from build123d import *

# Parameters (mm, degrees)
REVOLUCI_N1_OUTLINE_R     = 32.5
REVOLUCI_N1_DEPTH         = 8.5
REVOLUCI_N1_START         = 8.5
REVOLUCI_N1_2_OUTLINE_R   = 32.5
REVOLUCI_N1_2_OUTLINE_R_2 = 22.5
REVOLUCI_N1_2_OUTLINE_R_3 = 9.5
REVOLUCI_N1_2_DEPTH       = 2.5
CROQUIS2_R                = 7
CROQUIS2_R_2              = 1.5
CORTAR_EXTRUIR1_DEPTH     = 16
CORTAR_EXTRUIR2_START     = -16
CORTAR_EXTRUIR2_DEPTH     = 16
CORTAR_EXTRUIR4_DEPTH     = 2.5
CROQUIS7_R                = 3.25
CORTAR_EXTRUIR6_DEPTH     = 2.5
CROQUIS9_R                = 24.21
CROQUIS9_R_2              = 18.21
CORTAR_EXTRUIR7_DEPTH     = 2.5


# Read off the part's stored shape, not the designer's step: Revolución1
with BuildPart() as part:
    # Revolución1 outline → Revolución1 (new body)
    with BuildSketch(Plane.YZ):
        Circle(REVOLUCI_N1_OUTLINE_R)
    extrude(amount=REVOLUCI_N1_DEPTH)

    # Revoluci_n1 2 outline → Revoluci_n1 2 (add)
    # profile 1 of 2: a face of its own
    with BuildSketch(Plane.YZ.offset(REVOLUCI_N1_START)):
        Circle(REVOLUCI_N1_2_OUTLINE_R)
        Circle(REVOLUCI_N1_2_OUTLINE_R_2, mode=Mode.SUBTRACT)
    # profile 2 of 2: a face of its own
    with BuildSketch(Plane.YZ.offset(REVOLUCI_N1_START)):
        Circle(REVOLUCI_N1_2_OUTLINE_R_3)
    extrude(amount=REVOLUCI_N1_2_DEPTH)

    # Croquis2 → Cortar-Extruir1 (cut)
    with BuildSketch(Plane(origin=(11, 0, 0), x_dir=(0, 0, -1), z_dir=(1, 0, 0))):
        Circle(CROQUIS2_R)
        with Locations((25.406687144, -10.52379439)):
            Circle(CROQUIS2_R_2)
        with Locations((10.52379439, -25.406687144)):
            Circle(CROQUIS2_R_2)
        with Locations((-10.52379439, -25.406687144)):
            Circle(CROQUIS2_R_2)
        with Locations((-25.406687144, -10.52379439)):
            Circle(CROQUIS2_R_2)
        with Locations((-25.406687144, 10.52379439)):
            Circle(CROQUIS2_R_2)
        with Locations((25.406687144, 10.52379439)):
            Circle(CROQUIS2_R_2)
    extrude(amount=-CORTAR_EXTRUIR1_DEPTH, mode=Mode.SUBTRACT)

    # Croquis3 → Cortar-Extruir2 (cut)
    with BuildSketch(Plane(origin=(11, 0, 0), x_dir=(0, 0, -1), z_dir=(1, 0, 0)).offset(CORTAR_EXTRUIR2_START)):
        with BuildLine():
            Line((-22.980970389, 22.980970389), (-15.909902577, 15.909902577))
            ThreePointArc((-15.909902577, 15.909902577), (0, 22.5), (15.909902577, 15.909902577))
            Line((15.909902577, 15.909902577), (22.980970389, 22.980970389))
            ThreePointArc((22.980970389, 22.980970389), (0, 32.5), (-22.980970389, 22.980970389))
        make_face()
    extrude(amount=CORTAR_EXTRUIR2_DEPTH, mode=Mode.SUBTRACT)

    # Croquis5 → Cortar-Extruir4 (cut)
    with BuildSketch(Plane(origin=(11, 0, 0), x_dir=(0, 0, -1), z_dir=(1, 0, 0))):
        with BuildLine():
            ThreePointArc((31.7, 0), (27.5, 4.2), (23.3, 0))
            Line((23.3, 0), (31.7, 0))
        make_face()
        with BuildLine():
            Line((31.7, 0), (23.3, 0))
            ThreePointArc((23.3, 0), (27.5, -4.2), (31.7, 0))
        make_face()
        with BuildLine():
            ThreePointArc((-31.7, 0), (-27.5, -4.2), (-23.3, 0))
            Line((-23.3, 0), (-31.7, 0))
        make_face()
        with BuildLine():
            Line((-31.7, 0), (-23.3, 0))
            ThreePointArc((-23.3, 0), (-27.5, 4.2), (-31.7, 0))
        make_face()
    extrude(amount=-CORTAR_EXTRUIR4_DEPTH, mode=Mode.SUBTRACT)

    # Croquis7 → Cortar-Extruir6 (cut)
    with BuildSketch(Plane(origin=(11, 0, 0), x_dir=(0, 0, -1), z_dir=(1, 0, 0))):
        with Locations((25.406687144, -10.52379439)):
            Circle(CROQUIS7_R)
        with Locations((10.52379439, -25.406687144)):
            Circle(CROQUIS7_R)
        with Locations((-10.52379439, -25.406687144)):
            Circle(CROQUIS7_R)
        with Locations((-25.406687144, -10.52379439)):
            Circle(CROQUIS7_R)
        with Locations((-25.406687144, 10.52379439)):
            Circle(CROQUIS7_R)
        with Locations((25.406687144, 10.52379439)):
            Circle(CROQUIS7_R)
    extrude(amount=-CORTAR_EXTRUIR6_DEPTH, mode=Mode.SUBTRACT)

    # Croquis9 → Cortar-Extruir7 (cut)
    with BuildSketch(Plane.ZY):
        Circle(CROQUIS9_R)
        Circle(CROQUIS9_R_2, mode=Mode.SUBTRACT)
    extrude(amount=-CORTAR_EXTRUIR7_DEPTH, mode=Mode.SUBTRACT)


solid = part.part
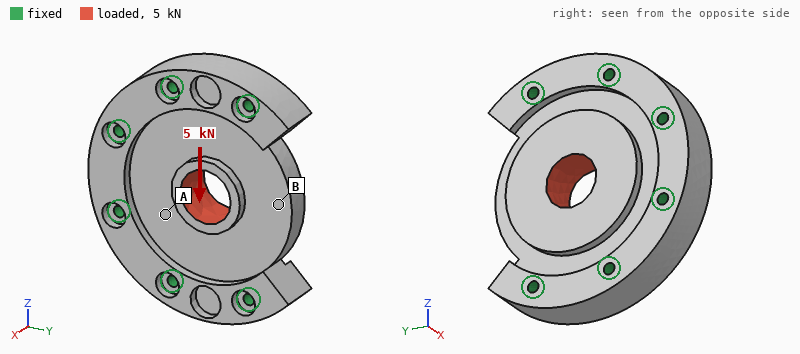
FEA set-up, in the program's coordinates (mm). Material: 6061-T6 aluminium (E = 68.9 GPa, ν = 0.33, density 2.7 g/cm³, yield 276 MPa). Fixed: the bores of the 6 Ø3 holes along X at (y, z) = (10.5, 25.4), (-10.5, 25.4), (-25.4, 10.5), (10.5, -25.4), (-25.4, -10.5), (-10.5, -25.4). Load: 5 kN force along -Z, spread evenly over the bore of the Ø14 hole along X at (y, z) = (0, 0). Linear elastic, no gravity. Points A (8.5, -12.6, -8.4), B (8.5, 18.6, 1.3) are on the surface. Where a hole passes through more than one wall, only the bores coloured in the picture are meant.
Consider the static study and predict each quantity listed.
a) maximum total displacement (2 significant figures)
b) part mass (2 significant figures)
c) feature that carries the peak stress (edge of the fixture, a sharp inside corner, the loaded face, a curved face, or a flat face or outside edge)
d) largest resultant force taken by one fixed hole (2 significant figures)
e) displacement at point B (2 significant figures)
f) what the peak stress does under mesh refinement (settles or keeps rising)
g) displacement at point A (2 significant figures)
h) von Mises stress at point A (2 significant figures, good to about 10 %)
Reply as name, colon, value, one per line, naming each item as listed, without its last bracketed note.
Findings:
maximum total displacement: 6.6 µm
part mass: 64 g
feature that carries the peak stress: edge of the fixture
largest resultant force taken by one fixed hole: 1.2 kN
displacement at point B: 2.4 µm
what the peak stress does under mesh refinement: keeps rising
displacement at point A: 1.9 µm
von Mises stress at point A: 9.1 MPa
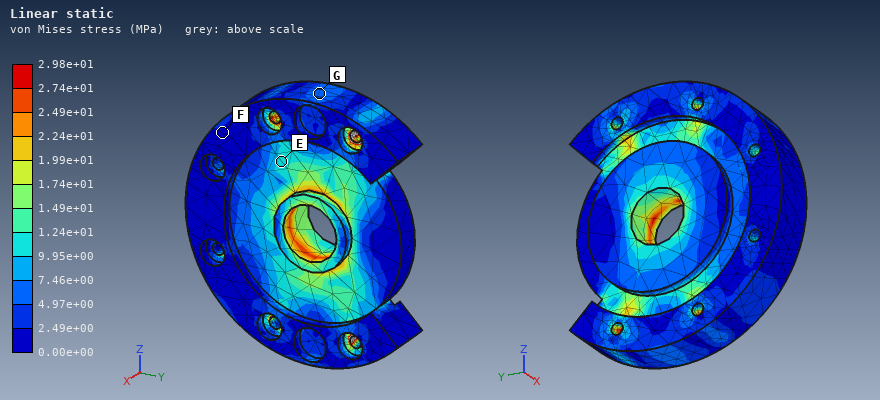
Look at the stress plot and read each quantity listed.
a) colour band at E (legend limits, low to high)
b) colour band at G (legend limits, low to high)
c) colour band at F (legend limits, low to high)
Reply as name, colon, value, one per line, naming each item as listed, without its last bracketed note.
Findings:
colour band at E: 9.95e+00 to 1.24e+01 MPa
colour band at G: 4.97e+00 to 7.46e+00 MPa
colour band at F: 0.00e+00 to 2.49e+00 MPa
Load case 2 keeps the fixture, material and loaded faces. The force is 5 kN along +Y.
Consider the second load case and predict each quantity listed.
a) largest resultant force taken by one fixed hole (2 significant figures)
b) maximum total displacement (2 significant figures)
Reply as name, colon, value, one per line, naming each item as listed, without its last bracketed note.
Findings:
largest resultant force taken by one fixed hole: 1.3 kN
maximum total displacement: 11 µm
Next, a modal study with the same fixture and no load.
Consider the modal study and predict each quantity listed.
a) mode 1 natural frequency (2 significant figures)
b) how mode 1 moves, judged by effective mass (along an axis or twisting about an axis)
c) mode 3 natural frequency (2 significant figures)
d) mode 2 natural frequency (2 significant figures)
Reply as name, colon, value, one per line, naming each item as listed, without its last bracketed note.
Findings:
mode 1 natural frequency: 12 kHz
how mode 1 moves, judged by effective mass: along X
mode 3 natural frequency: 28 kHz
mode 2 natural frequency: 22 kHz
